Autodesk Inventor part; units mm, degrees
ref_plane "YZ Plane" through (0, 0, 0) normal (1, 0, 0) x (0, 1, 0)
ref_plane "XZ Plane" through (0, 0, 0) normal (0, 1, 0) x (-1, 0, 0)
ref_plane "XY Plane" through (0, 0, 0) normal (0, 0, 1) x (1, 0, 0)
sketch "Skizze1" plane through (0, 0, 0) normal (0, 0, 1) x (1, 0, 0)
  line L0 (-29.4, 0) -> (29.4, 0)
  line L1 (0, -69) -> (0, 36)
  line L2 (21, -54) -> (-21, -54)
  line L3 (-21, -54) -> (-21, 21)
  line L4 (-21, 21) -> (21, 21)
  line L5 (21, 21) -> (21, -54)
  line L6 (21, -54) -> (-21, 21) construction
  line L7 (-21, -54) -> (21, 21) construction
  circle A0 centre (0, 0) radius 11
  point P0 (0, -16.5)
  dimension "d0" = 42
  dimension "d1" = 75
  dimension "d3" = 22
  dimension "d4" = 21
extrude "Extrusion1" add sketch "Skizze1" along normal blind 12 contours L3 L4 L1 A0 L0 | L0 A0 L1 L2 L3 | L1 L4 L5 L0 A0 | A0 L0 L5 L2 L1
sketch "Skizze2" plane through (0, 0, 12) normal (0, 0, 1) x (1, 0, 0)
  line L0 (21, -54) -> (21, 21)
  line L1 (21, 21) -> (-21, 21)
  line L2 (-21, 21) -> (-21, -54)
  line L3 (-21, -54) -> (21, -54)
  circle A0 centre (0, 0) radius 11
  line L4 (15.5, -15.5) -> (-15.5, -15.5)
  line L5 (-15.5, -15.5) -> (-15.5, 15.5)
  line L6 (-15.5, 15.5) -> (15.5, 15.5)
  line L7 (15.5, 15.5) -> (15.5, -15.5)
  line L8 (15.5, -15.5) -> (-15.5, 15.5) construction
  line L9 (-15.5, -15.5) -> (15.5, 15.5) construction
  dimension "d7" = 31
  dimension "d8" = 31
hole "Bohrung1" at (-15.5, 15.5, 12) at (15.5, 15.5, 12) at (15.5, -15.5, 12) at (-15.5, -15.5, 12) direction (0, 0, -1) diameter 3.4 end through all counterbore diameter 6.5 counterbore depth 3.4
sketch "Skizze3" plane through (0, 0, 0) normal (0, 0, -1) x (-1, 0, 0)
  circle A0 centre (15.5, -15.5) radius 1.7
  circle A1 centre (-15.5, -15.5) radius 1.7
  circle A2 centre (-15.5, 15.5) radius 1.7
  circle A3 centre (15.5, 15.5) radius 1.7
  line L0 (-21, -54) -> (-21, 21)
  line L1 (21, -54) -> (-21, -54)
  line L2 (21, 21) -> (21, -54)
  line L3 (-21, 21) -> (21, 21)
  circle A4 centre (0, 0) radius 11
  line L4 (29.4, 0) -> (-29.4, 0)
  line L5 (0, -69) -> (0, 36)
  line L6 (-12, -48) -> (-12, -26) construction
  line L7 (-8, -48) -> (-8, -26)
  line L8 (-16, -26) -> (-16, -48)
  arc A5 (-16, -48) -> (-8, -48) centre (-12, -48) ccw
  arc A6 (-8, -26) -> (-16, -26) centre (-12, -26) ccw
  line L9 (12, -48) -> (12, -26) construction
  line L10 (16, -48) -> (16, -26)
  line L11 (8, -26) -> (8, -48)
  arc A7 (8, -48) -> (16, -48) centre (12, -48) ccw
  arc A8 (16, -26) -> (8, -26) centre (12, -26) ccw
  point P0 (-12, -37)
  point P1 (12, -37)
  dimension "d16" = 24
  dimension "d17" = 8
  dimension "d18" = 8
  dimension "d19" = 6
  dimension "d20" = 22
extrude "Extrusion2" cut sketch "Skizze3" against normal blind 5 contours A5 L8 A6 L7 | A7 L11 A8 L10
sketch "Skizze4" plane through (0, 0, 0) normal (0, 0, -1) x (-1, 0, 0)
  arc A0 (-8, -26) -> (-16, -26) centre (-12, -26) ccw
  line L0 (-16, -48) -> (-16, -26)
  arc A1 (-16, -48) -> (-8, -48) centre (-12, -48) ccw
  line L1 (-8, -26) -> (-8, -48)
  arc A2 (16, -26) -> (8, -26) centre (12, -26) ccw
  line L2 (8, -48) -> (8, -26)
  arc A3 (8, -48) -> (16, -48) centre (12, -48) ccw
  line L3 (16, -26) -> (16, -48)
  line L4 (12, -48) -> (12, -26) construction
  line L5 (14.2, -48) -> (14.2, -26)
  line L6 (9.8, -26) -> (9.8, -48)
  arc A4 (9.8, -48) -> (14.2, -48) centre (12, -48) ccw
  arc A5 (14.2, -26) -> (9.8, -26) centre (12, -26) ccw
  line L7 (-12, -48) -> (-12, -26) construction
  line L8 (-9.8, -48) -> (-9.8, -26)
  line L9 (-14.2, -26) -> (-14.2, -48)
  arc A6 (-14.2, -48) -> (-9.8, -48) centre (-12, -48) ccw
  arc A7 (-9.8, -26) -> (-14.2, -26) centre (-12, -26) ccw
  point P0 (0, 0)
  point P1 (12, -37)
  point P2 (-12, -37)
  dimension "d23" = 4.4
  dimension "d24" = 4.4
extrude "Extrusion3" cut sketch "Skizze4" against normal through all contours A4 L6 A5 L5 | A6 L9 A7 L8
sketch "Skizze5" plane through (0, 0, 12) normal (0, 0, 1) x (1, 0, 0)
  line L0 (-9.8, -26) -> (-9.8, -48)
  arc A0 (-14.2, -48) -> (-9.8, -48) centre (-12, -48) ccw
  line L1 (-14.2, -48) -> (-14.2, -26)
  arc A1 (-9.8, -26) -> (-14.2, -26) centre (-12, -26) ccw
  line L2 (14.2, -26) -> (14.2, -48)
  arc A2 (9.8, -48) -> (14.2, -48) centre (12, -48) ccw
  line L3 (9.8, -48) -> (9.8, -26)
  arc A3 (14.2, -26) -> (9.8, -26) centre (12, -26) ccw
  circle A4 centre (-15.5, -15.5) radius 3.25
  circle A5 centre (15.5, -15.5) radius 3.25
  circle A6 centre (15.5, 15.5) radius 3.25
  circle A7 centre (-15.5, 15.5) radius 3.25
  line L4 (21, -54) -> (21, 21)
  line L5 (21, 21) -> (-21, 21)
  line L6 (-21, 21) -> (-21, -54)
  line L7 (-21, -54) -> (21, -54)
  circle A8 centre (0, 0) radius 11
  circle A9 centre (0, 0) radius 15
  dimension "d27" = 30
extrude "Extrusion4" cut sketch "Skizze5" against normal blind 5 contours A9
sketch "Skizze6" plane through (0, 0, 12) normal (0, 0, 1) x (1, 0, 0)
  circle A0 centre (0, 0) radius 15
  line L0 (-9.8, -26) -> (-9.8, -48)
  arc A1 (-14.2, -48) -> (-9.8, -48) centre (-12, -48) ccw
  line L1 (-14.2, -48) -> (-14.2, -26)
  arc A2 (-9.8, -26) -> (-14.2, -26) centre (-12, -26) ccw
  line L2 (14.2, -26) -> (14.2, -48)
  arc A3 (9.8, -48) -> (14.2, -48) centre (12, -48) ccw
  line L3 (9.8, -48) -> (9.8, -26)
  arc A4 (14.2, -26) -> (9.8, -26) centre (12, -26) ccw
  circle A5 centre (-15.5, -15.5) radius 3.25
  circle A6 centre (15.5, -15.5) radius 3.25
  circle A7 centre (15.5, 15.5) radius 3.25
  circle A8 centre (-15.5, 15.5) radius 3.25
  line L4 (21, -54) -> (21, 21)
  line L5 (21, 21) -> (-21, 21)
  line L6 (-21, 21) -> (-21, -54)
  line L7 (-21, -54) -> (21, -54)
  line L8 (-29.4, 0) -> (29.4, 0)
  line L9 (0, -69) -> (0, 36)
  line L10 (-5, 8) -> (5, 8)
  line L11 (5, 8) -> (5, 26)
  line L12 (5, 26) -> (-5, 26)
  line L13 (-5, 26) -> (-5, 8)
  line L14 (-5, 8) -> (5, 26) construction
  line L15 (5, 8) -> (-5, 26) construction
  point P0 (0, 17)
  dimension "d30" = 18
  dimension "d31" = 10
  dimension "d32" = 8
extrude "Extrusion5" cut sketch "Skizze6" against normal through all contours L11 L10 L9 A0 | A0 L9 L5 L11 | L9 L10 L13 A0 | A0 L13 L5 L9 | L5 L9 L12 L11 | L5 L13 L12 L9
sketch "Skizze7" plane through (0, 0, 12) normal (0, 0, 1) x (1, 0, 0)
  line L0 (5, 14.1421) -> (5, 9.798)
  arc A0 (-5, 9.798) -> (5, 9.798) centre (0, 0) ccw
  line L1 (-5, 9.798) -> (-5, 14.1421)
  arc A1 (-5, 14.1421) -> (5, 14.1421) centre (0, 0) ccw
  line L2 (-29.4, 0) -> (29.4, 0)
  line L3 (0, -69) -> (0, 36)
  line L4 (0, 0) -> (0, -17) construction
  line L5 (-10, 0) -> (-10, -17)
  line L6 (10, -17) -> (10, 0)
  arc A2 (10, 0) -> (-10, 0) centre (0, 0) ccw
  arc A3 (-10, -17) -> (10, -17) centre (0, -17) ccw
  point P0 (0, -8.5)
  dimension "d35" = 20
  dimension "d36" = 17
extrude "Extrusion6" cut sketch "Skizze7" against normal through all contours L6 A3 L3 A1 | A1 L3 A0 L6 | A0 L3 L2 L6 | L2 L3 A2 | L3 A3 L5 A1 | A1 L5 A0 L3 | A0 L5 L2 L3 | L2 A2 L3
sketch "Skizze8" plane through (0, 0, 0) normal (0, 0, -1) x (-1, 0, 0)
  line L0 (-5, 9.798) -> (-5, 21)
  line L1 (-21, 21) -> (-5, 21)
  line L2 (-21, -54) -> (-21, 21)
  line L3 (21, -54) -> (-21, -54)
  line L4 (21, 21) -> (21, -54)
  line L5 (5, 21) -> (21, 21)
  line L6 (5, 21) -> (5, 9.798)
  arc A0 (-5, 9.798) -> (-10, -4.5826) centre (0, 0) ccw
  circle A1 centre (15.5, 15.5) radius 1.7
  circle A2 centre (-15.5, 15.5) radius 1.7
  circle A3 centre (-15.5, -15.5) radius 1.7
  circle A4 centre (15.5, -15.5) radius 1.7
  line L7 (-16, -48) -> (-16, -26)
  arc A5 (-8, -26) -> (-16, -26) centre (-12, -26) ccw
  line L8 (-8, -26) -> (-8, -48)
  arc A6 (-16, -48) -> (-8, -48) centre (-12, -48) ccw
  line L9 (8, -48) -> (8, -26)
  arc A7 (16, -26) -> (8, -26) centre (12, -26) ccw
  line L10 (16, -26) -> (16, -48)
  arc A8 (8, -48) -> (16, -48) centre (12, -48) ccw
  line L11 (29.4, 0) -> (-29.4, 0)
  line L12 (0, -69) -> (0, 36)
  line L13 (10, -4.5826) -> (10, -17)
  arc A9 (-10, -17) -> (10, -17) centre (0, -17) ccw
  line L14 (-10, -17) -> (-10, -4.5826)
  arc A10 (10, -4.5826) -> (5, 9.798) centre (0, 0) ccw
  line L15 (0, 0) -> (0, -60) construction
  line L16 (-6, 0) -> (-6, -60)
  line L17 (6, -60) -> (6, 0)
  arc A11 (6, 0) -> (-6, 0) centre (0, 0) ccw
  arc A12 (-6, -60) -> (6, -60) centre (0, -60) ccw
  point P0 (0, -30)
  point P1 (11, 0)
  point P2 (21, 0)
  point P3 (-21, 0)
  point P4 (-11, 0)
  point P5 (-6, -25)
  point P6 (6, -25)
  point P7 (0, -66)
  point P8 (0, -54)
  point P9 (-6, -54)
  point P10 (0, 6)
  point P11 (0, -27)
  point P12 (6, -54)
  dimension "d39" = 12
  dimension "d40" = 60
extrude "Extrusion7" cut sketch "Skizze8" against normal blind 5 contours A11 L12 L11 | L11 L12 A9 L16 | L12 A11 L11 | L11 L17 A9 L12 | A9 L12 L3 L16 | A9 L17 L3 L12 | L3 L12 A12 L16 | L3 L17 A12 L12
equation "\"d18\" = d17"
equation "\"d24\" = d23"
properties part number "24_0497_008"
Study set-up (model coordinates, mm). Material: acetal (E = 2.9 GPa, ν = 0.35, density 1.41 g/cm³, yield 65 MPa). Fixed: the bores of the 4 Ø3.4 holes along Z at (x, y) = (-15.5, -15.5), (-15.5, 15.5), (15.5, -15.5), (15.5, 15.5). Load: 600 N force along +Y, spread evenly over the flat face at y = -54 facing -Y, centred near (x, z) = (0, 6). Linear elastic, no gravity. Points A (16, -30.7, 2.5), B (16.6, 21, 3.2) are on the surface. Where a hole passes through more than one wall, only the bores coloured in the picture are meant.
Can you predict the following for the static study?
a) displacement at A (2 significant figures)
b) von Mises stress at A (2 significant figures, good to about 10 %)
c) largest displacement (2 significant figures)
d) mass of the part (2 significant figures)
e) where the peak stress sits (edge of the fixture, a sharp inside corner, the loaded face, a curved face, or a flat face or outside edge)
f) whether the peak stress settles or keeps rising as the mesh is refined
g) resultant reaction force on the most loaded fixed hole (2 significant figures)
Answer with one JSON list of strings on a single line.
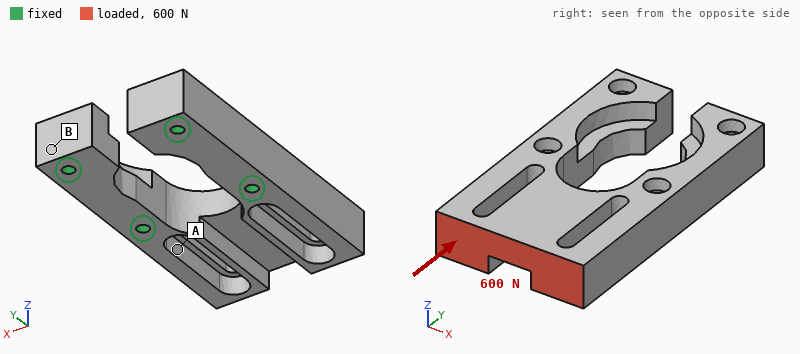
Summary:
["18 µm", "2.8 MPa", "61 µm", "30 g", "edge of the fixture", "keeps rising", "280 N"]
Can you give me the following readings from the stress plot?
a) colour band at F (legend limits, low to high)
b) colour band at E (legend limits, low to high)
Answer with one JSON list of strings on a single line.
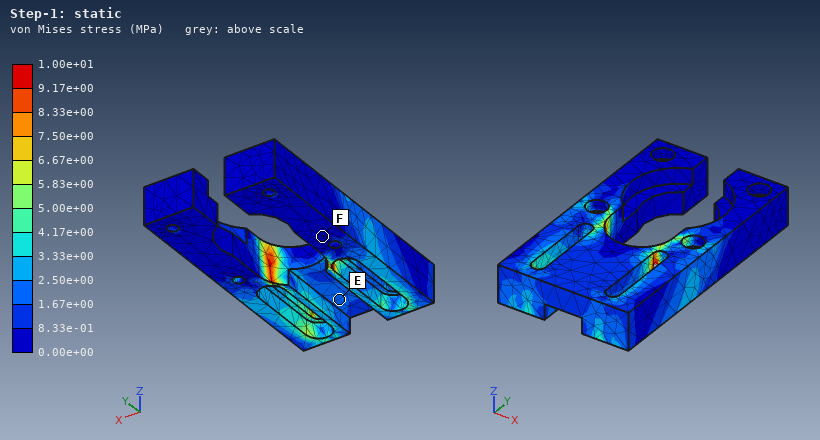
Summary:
["0.00e+00 to 8.33e-01 MPa", "1.67e+00 to 2.50e+00 MPa"]
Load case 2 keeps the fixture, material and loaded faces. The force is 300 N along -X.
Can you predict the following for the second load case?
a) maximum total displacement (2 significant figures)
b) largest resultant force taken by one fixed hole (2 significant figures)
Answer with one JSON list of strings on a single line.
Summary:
["0.27 mm", "340 N"]
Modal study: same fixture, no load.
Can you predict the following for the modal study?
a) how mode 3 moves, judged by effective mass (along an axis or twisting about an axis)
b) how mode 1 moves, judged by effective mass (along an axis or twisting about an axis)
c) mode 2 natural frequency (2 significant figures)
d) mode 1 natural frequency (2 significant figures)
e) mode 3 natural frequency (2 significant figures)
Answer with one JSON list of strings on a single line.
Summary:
["along X", "along Z", "2000 Hz", "1200 Hz", "2600 Hz"]
